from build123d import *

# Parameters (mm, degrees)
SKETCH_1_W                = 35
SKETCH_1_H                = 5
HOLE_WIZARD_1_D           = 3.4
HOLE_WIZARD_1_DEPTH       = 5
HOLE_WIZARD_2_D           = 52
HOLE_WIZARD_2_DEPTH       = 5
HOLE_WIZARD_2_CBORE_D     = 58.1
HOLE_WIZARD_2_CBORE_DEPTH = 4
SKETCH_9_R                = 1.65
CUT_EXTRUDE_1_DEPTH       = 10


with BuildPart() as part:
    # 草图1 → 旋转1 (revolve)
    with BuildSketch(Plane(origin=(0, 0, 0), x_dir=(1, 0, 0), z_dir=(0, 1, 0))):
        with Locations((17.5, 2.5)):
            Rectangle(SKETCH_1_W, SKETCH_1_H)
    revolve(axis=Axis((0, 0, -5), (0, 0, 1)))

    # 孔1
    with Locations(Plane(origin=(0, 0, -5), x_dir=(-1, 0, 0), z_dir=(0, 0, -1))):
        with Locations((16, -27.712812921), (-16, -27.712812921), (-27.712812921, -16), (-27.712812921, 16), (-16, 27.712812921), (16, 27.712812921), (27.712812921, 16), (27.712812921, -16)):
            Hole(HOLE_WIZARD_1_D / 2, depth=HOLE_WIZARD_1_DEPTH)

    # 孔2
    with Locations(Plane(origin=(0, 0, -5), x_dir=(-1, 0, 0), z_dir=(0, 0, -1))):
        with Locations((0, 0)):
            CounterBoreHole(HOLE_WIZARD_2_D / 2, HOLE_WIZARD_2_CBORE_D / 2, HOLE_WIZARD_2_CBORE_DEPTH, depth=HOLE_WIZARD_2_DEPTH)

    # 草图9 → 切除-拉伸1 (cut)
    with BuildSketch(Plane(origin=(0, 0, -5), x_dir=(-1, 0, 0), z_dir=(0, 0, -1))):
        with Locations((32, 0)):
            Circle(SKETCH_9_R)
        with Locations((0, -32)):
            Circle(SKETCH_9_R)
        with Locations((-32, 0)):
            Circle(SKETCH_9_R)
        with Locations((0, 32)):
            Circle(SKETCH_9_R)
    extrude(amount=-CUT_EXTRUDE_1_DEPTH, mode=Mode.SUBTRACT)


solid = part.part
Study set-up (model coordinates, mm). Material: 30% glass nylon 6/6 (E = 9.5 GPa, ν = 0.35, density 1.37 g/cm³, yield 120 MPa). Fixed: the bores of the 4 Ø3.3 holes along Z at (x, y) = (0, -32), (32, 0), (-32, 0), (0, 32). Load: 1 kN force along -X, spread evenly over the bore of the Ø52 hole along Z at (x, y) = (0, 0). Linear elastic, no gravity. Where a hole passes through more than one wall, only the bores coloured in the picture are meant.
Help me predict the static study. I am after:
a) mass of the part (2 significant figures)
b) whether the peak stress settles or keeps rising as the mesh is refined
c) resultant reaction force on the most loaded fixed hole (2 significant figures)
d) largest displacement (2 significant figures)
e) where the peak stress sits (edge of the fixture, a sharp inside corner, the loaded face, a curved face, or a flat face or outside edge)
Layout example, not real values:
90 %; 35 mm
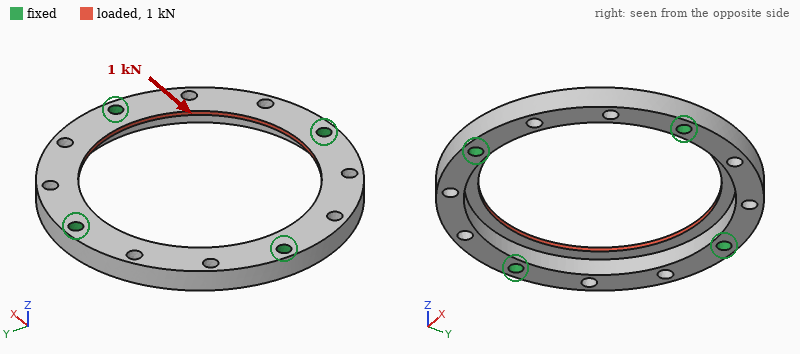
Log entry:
8.2 g; keeps rising; 350 N; 44 µm; edge of the fixture
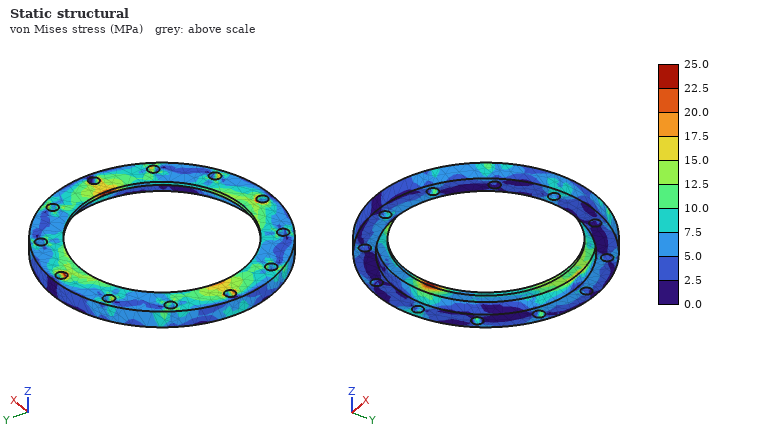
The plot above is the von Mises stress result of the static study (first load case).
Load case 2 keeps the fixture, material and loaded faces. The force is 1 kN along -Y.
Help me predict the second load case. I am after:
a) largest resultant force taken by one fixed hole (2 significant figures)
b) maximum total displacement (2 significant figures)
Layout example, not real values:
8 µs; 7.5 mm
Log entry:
350 N; 44 µm
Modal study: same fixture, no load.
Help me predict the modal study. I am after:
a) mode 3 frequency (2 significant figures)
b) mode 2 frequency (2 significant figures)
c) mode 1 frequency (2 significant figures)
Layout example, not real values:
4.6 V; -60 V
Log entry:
5200 Hz; 5200 Hz; 5100 Hz
